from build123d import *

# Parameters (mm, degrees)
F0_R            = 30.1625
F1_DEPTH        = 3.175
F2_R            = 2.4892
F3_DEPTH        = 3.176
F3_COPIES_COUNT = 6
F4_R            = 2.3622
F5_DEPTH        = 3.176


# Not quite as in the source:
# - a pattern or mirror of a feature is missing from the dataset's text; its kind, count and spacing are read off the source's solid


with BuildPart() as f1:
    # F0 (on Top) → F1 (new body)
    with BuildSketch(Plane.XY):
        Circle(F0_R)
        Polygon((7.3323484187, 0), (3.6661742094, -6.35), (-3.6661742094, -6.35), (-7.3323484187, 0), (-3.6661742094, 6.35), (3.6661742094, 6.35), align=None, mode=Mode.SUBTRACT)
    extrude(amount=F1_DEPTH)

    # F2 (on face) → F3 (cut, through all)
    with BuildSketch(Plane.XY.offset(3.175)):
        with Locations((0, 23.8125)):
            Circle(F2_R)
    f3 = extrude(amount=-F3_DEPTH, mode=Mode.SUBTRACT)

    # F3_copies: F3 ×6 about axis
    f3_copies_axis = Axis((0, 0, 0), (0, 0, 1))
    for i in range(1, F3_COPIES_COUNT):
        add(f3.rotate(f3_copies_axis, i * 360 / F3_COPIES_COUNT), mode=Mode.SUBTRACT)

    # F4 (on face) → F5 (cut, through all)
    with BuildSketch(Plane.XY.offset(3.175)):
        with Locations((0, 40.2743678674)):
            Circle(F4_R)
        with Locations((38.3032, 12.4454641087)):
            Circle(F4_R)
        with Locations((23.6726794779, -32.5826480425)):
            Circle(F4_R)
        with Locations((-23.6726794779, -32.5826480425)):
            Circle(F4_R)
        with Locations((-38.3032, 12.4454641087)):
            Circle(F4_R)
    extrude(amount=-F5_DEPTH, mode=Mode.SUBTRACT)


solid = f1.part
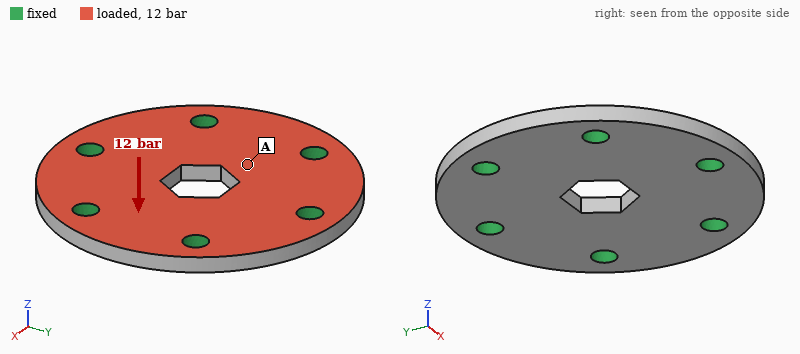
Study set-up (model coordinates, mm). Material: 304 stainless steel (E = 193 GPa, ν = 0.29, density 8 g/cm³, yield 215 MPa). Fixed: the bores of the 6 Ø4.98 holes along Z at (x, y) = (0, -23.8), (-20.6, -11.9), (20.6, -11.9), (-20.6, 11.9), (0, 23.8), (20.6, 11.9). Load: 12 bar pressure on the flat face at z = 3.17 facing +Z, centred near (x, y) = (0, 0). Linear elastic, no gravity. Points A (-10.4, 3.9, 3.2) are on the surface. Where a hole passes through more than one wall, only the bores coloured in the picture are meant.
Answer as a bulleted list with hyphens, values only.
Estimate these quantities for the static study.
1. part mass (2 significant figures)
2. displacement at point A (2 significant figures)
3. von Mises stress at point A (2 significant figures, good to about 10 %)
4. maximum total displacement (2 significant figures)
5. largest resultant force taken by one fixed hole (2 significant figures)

- 66 g
- 6.4 µm
- 14 MPa
- 9.5 µm
- 520 N
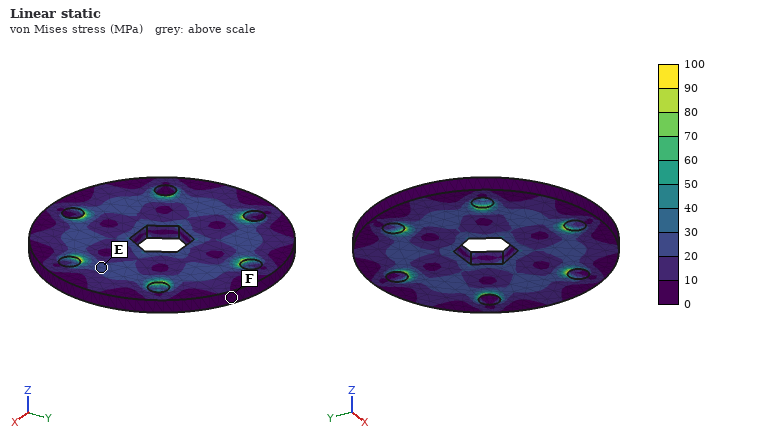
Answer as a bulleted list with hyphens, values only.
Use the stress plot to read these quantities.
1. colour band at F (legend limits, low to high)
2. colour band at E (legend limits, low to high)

- 0 to 10 MPa
- 20 to 30 MPa
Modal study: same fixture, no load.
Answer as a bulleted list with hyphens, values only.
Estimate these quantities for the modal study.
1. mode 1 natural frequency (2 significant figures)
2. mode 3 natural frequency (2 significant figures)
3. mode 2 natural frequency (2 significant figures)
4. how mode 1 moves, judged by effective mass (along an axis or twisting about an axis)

- 14 kHz
- 23 kHz
- 23 kHz
- along Z
